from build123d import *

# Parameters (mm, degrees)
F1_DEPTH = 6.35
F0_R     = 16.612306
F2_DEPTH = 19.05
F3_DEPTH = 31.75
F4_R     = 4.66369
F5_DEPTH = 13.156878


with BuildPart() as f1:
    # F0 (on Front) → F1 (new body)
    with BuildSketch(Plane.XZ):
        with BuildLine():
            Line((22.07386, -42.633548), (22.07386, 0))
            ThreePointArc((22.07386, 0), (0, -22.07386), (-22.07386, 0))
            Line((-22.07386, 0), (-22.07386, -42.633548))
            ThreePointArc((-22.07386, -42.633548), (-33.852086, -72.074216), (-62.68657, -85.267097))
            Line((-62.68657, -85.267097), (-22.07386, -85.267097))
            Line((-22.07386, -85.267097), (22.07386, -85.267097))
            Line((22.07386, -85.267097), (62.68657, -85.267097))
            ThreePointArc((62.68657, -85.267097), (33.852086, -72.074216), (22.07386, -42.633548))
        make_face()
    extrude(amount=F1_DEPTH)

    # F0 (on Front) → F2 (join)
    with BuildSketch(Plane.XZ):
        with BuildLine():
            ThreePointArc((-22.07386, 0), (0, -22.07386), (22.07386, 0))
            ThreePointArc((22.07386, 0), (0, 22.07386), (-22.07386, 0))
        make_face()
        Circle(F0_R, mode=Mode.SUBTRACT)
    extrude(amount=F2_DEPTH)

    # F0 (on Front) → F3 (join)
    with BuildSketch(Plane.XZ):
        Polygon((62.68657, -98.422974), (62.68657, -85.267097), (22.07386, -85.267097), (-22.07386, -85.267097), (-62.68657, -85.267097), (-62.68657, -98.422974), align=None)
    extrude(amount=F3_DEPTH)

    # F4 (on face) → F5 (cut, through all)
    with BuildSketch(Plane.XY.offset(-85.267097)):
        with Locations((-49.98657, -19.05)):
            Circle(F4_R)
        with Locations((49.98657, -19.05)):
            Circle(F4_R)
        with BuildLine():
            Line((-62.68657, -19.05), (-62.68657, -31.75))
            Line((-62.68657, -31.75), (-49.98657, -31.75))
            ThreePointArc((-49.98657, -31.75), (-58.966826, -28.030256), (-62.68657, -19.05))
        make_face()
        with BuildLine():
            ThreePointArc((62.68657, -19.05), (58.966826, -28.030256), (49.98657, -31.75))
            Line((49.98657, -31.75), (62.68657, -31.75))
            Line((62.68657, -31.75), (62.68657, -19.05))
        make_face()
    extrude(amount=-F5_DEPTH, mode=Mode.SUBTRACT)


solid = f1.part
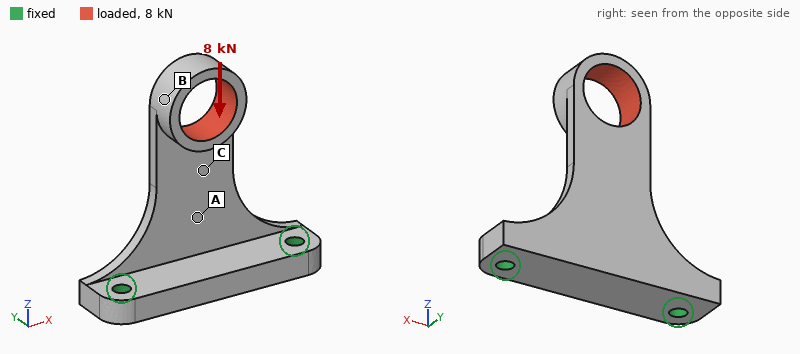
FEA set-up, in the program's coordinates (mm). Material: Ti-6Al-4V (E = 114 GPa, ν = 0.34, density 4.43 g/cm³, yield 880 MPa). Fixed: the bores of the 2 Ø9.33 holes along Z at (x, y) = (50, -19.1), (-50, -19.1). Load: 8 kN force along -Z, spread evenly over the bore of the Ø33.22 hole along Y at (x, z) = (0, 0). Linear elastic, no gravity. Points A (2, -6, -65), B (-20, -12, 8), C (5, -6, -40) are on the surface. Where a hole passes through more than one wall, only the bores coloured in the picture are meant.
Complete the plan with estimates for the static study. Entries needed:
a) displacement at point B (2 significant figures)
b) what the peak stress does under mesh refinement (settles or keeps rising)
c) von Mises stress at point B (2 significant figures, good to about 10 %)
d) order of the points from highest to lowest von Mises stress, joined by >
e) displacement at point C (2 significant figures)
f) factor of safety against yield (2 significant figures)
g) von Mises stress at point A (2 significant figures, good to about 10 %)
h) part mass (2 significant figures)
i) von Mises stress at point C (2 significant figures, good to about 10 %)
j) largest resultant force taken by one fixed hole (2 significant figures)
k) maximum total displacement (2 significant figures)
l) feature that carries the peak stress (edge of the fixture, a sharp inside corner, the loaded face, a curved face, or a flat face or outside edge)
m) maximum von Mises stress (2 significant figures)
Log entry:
1.6 mm
settles
35 MPa
C > A > B
0.37 mm
3.8
140 MPa
380 g
180 MPa
4.2 kN
2.1 mm
a curved face
230 MPa
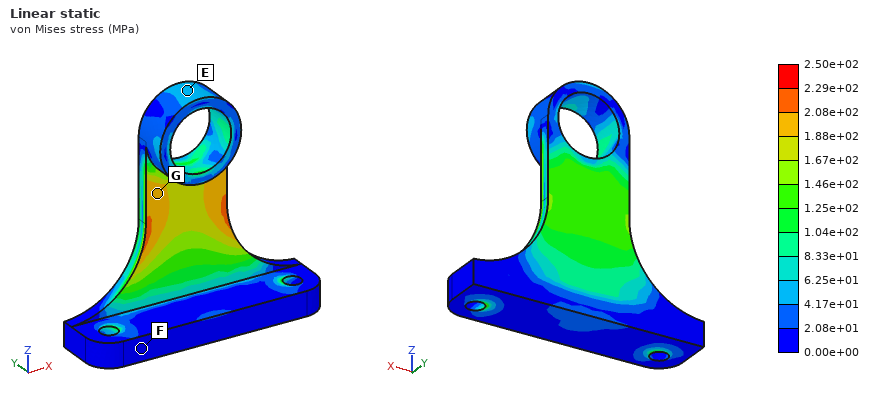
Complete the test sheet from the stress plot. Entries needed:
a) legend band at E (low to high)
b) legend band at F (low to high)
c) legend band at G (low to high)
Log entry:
4.17e+01 to 6.25e+01 MPa
0.00e+00 to 2.08e+01 MPa
1.88e+02 to 2.08e+02 MPa
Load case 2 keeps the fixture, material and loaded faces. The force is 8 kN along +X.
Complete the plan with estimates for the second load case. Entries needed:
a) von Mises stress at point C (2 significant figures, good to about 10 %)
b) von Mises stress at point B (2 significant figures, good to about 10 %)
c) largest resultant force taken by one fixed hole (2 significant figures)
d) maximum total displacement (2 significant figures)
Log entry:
210 MPa
83 MPa
9.3 kN
0.86 mm
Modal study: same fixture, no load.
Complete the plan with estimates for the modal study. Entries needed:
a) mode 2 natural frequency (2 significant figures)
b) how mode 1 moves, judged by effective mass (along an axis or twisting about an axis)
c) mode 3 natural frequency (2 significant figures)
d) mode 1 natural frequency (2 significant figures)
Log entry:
1900 Hz
along Y
2500 Hz
460 Hz
